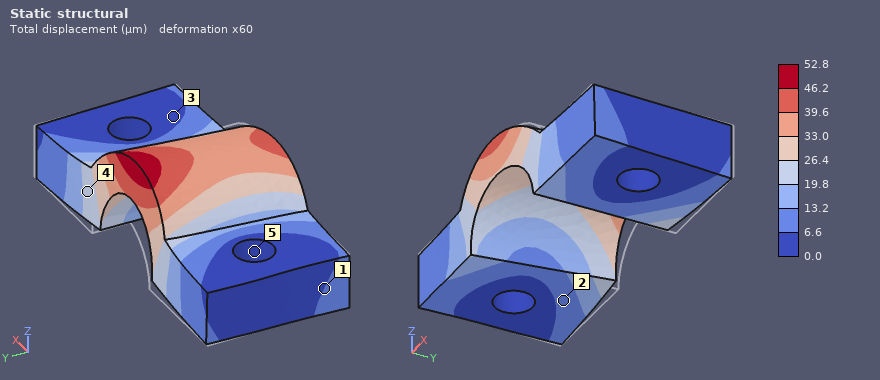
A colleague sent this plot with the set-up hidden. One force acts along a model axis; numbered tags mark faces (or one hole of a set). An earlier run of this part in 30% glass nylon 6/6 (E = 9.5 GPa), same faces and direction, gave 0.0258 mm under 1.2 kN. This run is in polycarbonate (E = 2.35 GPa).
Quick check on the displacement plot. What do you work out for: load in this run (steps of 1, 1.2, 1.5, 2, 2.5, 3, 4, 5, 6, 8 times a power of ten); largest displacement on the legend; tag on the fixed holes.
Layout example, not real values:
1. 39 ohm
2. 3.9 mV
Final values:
1. 600 N
2. 52.8 µm
3. 5
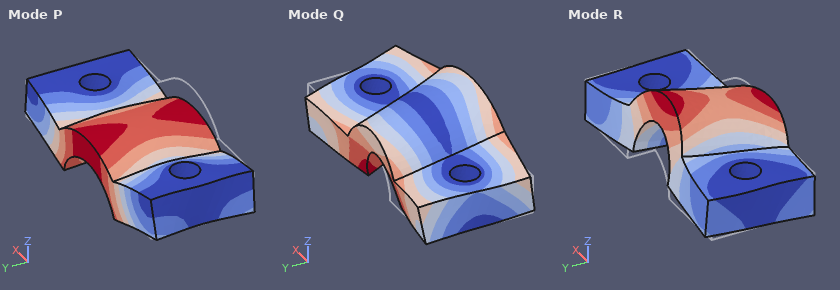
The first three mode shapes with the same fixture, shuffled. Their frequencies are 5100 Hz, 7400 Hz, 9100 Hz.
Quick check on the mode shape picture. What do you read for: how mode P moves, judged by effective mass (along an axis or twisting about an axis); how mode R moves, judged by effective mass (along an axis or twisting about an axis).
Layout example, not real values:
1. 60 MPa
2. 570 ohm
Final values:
1. along Z
2. along Y
